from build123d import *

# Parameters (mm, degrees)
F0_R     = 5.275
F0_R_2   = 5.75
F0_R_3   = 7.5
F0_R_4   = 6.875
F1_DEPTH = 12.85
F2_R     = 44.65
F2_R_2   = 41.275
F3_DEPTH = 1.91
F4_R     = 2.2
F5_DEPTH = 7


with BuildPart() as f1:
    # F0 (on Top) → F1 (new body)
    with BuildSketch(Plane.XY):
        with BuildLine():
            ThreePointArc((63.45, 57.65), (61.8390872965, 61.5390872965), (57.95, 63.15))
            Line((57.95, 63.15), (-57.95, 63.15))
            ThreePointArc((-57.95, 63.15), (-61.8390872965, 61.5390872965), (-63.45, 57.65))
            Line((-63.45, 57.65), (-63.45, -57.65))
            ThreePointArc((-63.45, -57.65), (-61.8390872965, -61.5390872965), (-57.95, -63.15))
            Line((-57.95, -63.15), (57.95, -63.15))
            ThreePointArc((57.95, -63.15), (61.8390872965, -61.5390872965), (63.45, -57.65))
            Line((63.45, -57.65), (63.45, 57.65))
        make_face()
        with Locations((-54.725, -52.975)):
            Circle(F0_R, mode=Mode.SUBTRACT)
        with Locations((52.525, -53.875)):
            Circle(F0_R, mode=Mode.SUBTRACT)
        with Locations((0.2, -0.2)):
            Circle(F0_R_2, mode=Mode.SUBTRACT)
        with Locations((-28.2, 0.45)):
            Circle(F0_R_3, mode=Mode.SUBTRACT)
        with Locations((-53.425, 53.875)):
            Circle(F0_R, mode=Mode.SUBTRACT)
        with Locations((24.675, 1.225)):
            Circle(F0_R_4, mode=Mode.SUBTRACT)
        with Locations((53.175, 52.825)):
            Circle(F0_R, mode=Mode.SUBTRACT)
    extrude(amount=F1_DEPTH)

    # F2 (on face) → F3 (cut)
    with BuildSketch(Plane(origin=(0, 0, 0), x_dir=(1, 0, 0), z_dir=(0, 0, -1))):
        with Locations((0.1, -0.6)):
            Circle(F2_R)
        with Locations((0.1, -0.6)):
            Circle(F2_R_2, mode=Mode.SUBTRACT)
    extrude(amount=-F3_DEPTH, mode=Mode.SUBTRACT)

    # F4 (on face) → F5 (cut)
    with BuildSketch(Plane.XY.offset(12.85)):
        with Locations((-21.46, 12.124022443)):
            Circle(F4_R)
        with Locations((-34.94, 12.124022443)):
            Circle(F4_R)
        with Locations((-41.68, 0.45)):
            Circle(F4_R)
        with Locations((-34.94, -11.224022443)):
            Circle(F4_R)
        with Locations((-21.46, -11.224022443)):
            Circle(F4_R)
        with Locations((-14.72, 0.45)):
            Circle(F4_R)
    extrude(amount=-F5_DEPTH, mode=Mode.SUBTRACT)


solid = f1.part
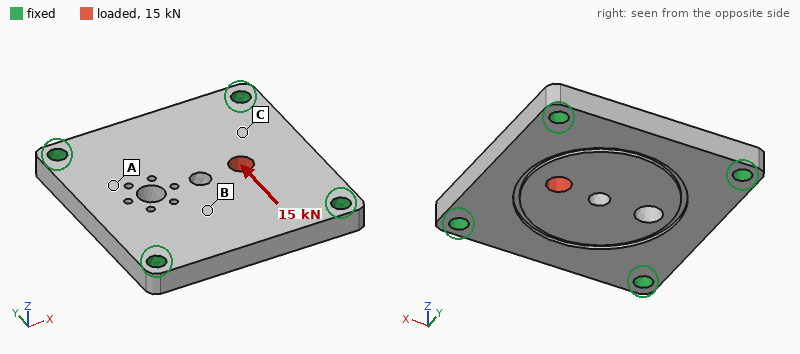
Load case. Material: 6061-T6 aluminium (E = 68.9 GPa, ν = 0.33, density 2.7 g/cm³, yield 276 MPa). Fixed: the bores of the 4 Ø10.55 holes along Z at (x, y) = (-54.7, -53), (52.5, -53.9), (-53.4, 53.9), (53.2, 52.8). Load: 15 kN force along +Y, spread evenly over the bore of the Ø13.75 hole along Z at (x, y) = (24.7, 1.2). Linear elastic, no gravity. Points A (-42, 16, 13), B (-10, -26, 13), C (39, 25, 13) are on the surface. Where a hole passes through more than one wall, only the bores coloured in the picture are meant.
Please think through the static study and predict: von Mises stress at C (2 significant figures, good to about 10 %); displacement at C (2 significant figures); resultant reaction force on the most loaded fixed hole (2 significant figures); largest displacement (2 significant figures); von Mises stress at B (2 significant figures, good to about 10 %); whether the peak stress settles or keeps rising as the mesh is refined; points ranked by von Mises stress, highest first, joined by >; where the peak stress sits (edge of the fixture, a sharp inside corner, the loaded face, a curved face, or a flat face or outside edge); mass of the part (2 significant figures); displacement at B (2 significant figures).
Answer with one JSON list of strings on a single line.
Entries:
["16 MPa", "7.7 µm", "5.8 kN", "16 µm", "6.0 MPa", "keeps rising", "C > B > A", "a sharp inside corner", "520 g", "7.0 µm"]
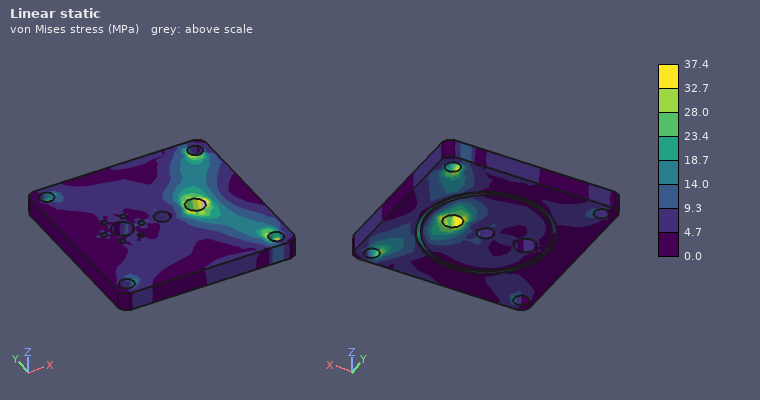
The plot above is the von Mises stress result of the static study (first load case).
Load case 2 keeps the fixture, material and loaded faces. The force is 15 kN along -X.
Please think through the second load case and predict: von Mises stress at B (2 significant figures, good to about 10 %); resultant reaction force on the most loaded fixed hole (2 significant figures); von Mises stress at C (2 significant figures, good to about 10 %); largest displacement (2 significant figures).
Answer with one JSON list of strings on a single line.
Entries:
["11 MPa", "4.8 kN", "14 MPa", "21 µm"]
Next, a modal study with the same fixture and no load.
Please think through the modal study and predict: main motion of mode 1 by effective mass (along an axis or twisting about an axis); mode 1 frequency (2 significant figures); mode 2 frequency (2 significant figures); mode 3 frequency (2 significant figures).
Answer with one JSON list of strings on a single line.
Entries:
["along Z", "3700 Hz", "6100 Hz", "6200 Hz"]
